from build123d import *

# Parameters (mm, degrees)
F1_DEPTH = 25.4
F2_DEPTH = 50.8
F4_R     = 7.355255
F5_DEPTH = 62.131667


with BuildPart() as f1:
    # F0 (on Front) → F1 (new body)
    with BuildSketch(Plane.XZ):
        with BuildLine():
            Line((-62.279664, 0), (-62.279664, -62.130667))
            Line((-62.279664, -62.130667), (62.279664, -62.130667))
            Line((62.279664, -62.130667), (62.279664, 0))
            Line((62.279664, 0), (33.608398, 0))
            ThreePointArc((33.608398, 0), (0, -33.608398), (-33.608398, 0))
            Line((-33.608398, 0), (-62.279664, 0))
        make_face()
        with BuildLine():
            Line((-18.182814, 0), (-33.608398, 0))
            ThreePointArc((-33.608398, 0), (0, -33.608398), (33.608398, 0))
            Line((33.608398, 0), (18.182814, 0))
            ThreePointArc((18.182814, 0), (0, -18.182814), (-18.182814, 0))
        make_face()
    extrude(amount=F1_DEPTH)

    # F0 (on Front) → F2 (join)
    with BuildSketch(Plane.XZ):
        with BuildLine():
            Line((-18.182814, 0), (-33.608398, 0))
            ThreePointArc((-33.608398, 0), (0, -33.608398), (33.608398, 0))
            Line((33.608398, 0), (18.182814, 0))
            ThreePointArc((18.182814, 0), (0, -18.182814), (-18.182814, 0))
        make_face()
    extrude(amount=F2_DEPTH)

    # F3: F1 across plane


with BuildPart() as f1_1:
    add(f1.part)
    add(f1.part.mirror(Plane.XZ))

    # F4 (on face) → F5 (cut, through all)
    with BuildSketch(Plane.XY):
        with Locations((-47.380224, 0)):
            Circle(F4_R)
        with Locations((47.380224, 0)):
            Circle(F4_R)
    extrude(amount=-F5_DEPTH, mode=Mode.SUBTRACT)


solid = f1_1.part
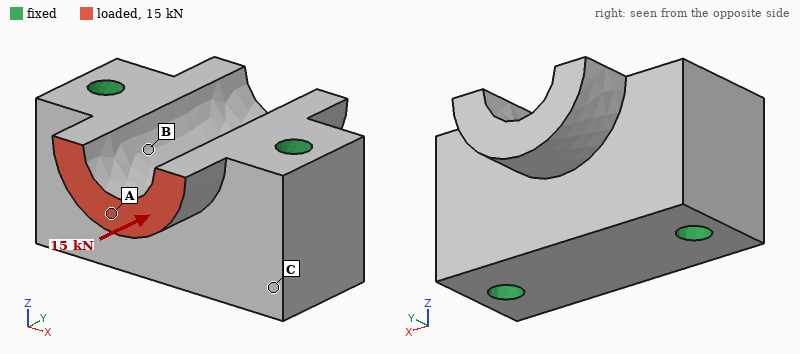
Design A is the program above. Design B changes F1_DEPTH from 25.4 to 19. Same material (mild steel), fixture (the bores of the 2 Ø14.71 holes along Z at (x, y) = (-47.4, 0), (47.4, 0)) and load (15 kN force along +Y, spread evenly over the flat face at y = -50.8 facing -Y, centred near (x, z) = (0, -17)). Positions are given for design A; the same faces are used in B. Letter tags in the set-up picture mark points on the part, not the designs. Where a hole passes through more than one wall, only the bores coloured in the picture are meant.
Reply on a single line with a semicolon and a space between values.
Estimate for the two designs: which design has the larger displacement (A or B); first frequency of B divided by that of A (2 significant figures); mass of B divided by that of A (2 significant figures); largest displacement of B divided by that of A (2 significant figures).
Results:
B; 0.81; 0.81; 1.1
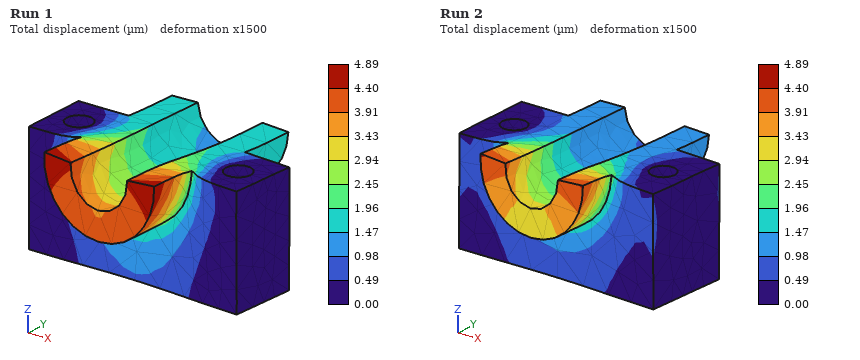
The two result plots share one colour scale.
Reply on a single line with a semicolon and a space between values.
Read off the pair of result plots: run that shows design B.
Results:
Run 1
